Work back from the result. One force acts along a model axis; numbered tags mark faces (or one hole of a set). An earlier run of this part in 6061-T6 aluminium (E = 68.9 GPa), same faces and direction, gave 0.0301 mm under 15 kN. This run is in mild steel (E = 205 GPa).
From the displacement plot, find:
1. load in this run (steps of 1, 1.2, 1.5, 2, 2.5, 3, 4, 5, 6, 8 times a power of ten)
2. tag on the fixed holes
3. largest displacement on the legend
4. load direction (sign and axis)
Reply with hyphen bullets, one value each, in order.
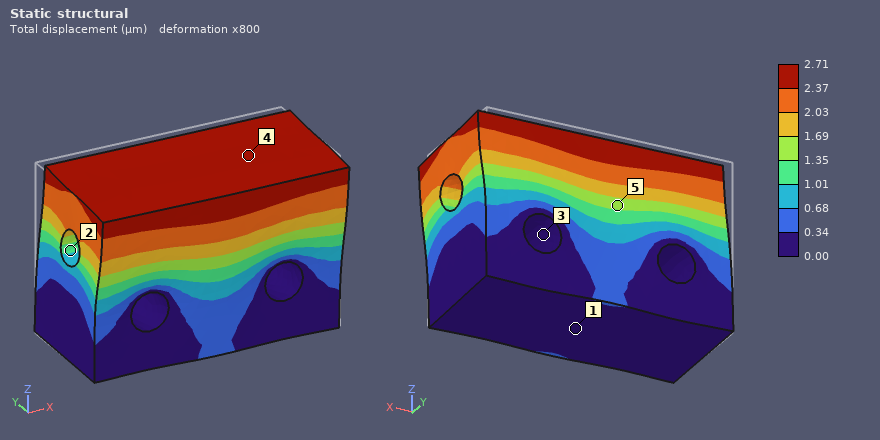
- 4 kN
- 3
- 2.71 µm
- -Y
